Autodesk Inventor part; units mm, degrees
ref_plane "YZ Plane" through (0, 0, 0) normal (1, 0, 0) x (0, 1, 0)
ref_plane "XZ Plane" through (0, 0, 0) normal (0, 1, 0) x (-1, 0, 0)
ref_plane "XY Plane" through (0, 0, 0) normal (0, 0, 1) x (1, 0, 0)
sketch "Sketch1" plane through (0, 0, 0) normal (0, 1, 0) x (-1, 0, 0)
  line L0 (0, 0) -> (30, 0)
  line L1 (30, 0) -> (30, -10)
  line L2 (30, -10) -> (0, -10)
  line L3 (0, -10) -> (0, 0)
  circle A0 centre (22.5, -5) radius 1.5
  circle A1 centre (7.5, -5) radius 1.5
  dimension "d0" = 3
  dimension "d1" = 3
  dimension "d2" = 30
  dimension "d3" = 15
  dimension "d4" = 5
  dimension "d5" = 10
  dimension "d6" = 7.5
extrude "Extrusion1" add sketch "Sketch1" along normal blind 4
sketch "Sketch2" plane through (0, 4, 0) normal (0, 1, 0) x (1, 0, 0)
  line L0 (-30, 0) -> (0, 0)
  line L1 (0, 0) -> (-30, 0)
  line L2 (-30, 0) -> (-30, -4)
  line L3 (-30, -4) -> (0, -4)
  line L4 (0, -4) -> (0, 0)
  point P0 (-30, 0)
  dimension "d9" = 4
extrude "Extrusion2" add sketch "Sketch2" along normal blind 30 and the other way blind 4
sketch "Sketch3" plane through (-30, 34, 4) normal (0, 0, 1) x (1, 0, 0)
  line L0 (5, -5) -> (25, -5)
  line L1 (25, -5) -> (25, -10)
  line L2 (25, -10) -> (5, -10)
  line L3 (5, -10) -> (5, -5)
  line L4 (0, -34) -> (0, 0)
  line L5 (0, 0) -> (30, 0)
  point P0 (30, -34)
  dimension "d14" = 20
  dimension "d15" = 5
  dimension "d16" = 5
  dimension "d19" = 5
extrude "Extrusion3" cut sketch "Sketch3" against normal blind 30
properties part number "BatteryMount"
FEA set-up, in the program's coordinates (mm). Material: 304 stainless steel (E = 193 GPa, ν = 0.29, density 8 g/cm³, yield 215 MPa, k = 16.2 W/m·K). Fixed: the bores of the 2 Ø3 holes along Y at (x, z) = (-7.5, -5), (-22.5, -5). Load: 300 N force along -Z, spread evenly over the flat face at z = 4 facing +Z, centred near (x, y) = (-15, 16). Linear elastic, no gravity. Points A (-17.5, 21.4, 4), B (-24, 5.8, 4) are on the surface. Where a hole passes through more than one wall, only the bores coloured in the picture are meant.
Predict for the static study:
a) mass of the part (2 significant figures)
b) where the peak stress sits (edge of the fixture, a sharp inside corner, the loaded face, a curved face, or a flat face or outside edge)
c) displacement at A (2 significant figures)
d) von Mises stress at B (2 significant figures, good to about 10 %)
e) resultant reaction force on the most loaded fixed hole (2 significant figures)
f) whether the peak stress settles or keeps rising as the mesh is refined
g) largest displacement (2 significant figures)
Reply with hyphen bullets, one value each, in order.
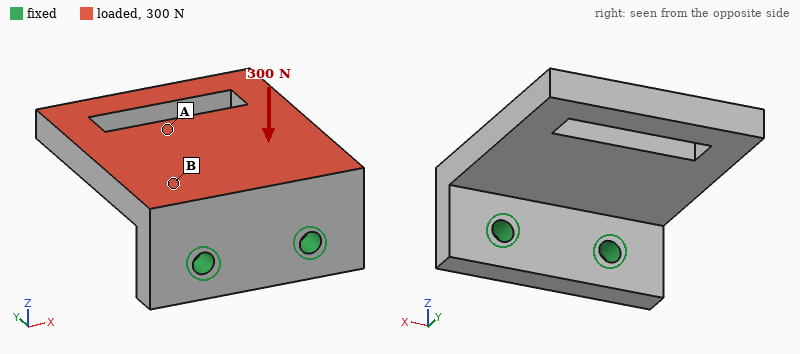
- 39 g
- edge of the fixture
- 33 µm
- 38 MPa
- 150 N
- keeps rising
- 63 µm
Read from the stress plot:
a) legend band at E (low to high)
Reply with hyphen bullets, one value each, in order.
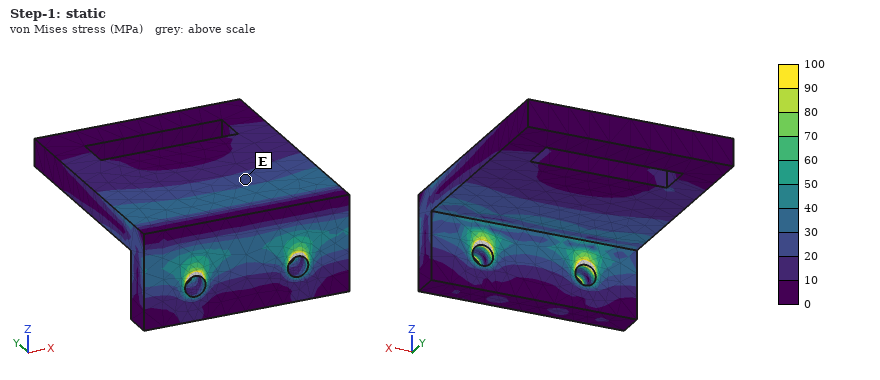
- 20 to 30 MPa
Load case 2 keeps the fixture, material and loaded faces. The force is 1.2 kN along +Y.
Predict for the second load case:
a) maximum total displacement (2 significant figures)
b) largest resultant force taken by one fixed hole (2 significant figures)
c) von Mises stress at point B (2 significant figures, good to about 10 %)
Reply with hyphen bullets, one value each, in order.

- 78 µm
- 600 N
- 33 MPa
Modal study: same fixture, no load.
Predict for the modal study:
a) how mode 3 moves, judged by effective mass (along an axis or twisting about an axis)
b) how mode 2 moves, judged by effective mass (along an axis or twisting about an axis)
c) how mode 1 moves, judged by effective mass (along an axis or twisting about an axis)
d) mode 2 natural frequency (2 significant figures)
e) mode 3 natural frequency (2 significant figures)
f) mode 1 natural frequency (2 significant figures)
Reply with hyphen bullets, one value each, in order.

- along X
- along X
- along Z
- 6100 Hz
- 7800 Hz
- 2500 Hz
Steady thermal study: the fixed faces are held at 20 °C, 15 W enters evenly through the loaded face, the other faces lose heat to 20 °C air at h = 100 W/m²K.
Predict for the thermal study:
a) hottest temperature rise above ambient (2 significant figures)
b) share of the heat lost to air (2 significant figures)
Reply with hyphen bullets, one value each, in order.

- 62 K
- 54 %
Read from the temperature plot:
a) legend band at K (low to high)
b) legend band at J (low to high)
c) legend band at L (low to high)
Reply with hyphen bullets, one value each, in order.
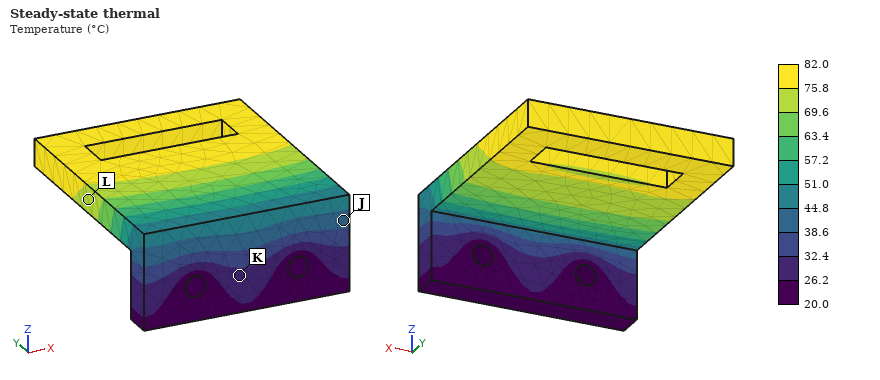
- 26.2 to 32.4 °C
- 38.6 to 44.8 °C
- 69.6 to 75.8 °C
